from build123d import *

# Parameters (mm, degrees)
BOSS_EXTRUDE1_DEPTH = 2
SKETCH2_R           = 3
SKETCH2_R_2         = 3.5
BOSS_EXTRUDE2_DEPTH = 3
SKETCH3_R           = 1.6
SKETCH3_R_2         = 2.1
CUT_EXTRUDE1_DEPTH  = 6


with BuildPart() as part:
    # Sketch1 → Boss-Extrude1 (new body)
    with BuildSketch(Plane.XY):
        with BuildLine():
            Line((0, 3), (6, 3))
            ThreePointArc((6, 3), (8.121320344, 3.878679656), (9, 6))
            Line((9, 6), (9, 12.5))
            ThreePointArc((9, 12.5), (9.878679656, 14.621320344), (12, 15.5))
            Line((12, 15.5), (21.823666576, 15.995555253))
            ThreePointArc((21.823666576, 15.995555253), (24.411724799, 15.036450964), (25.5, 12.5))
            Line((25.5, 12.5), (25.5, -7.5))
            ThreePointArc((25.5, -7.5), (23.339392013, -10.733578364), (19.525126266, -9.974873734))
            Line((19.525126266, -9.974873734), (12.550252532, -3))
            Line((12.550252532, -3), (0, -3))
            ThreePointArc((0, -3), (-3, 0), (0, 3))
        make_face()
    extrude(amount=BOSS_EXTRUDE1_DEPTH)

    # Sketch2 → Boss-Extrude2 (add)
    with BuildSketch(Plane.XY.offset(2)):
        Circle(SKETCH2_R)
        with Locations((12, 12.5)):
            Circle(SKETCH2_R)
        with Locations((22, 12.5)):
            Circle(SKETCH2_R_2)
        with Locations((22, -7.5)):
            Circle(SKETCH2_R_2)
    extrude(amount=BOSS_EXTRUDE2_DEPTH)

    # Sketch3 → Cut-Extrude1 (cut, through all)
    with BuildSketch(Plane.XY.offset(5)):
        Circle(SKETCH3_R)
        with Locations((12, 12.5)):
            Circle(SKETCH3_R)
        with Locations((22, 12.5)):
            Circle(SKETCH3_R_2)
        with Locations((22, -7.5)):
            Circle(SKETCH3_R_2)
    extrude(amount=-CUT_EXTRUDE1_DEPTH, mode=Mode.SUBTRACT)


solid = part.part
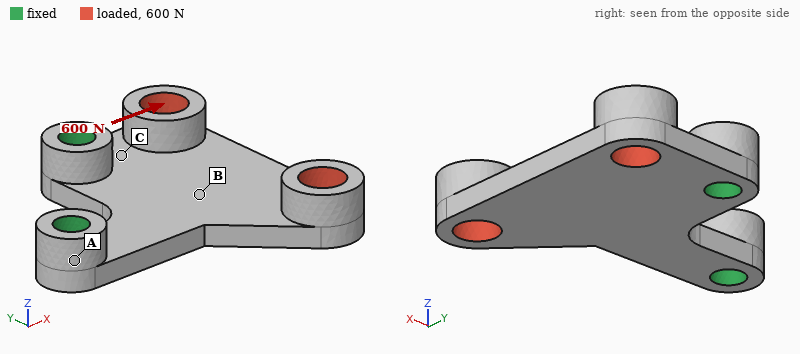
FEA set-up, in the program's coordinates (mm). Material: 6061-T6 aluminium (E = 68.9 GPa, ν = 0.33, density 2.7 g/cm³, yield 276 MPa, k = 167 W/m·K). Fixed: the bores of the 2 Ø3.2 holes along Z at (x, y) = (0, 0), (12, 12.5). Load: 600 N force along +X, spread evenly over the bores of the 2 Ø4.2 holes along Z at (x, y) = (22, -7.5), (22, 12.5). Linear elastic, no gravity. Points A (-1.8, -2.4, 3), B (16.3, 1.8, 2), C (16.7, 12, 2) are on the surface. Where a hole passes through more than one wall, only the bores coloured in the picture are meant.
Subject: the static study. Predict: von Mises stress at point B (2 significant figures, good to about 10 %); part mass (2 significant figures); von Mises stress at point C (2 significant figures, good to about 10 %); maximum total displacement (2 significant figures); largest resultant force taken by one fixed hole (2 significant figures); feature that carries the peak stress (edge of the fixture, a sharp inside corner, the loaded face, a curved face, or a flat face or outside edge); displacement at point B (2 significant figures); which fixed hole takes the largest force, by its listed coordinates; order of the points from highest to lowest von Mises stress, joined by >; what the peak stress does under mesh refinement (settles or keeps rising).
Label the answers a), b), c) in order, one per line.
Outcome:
a) 54 MPa
b) 2.9 g
c) 93 MPa
d) 0.14 mm
e) 410 N
f) a sharp inside corner
g) 0.025 mm
h) (0, 0)
i) C > B > A
j) keeps rising
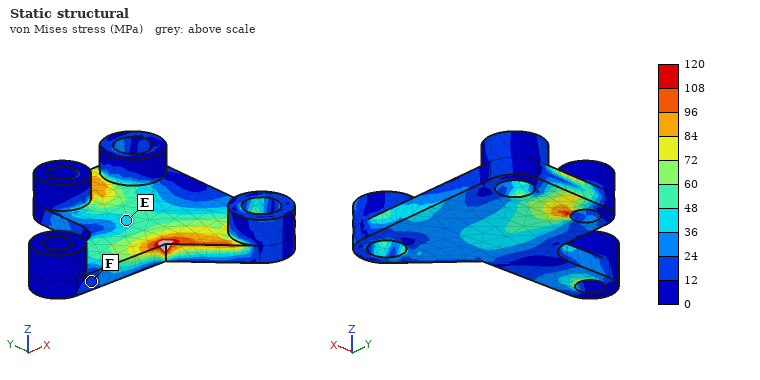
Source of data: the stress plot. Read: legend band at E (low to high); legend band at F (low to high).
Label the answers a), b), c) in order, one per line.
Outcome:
a) 36 to 48 MPa
b) 12 to 24 MPa
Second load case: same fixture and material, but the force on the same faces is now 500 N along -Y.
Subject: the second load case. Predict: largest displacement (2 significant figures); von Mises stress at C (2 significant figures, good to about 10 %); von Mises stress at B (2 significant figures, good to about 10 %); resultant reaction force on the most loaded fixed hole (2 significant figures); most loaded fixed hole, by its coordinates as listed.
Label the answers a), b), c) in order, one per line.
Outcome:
a) 0.15 mm
b) 84 MPa
c) 54 MPa
d) 590 N
e) (12, 12.5)
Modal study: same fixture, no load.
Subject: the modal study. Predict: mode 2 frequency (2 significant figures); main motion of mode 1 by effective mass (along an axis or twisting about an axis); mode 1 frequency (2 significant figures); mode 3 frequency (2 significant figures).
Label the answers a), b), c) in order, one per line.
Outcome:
a) 10000 Hz
b) along Z
c) 3700 Hz
d) 18 kHz
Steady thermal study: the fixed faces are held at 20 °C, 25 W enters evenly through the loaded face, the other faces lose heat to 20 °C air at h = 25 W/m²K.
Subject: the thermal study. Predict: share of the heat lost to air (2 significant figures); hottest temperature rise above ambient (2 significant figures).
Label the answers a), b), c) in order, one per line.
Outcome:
a) 3.7 %
b) 74 K
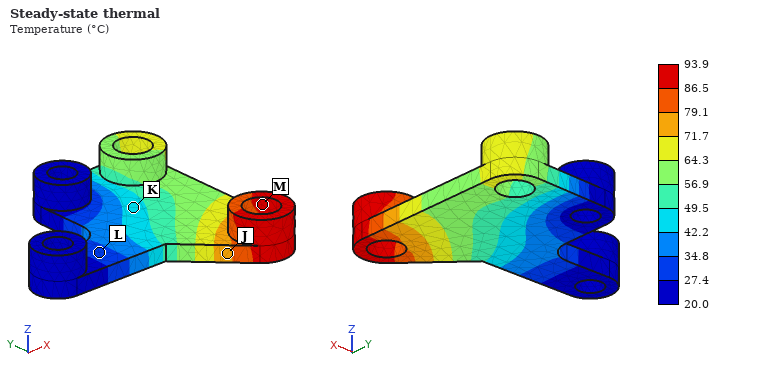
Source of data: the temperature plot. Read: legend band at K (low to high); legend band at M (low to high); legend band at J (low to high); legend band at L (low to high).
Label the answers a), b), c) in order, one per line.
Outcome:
a) 42.2 to 49.5 °C
b) 86.5 to 93.9 °C
c) 71.7 to 79.1 °C
d) 27.4 to 34.8 °C
